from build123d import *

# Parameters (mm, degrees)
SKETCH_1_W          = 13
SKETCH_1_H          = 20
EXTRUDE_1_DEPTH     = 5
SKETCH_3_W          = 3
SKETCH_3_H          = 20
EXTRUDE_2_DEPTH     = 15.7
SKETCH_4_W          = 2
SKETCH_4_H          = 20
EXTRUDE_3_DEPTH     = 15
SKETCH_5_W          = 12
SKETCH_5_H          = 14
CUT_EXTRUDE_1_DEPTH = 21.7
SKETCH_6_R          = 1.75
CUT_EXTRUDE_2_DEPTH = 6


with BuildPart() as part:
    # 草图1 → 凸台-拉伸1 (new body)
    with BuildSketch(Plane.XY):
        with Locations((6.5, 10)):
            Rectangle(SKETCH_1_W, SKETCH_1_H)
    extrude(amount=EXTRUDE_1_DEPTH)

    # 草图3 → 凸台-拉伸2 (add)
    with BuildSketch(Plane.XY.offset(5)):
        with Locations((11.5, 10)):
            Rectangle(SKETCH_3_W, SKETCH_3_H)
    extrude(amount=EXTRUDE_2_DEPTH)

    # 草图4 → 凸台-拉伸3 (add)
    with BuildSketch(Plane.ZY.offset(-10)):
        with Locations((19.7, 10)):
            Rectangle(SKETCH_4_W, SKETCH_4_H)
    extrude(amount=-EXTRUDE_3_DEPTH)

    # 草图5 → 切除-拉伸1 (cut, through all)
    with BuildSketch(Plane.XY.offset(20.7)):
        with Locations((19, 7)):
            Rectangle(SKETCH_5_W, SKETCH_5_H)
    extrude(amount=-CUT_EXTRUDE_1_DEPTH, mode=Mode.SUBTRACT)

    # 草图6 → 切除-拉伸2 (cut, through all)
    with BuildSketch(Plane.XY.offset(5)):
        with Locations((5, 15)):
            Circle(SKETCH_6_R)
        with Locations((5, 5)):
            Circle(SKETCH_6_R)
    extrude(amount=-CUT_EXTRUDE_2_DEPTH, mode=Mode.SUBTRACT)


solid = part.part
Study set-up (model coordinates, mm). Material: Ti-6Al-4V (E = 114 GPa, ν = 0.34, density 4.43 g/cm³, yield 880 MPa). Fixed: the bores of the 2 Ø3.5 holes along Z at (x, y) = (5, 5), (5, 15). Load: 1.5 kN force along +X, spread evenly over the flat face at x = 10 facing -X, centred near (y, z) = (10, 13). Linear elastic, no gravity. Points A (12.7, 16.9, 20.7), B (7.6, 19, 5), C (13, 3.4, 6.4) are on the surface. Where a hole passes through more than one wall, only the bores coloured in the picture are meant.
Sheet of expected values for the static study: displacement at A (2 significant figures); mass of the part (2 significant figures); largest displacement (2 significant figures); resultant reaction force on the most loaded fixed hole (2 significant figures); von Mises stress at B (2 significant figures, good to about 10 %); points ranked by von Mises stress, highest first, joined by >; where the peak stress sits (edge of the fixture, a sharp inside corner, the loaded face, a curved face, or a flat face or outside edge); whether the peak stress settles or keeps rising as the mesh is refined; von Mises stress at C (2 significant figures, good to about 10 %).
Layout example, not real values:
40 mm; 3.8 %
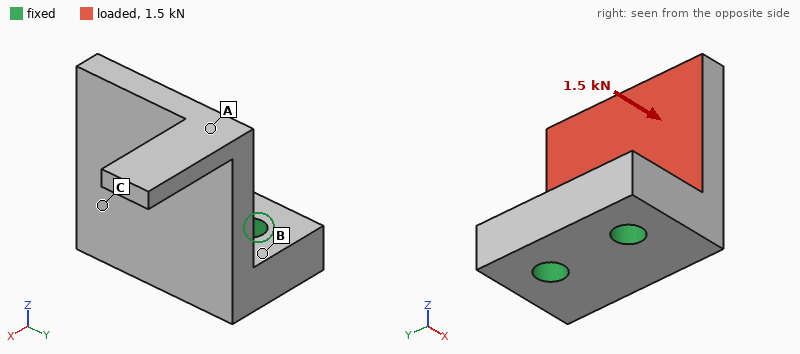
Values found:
0.25 mm; 10 g; 0.35 mm; 780 N; 120 MPa; C > B > A; edge of the fixture; keeps rising; 290 MPa
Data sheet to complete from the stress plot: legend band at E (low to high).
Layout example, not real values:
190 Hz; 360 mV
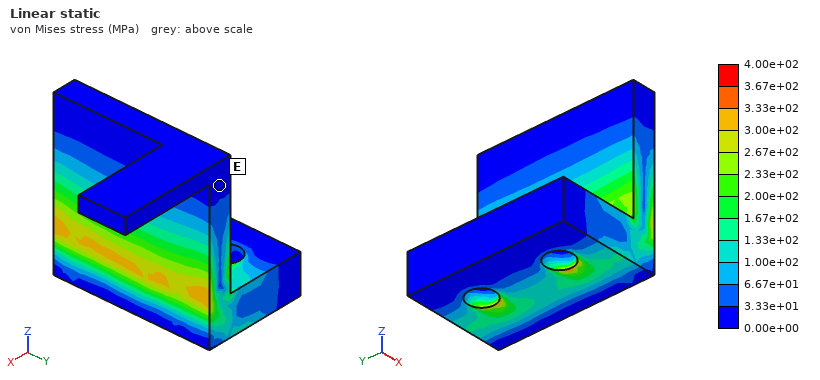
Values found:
0.00e+00 to 3.33e+01 MPa
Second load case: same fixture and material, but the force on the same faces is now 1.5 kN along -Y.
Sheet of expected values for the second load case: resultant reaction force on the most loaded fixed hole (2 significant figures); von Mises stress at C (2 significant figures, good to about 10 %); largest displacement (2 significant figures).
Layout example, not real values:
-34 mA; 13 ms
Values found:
1.4 kN; 34 MPa; 53 µm
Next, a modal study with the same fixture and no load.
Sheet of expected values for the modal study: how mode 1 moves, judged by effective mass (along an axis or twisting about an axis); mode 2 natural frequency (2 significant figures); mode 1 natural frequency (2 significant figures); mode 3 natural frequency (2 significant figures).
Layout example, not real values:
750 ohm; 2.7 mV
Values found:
along X; 9600 Hz; 5400 Hz; 10 kHz
